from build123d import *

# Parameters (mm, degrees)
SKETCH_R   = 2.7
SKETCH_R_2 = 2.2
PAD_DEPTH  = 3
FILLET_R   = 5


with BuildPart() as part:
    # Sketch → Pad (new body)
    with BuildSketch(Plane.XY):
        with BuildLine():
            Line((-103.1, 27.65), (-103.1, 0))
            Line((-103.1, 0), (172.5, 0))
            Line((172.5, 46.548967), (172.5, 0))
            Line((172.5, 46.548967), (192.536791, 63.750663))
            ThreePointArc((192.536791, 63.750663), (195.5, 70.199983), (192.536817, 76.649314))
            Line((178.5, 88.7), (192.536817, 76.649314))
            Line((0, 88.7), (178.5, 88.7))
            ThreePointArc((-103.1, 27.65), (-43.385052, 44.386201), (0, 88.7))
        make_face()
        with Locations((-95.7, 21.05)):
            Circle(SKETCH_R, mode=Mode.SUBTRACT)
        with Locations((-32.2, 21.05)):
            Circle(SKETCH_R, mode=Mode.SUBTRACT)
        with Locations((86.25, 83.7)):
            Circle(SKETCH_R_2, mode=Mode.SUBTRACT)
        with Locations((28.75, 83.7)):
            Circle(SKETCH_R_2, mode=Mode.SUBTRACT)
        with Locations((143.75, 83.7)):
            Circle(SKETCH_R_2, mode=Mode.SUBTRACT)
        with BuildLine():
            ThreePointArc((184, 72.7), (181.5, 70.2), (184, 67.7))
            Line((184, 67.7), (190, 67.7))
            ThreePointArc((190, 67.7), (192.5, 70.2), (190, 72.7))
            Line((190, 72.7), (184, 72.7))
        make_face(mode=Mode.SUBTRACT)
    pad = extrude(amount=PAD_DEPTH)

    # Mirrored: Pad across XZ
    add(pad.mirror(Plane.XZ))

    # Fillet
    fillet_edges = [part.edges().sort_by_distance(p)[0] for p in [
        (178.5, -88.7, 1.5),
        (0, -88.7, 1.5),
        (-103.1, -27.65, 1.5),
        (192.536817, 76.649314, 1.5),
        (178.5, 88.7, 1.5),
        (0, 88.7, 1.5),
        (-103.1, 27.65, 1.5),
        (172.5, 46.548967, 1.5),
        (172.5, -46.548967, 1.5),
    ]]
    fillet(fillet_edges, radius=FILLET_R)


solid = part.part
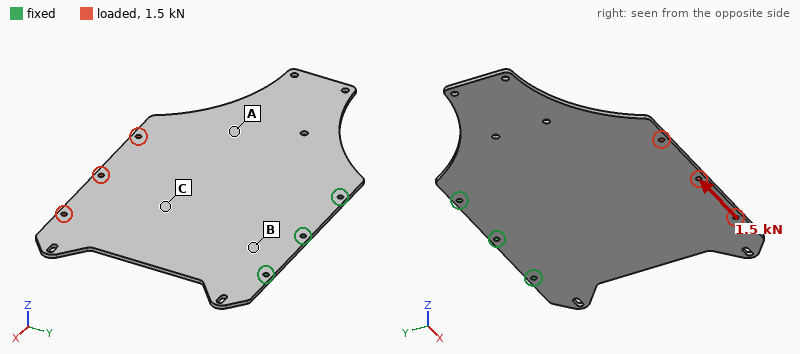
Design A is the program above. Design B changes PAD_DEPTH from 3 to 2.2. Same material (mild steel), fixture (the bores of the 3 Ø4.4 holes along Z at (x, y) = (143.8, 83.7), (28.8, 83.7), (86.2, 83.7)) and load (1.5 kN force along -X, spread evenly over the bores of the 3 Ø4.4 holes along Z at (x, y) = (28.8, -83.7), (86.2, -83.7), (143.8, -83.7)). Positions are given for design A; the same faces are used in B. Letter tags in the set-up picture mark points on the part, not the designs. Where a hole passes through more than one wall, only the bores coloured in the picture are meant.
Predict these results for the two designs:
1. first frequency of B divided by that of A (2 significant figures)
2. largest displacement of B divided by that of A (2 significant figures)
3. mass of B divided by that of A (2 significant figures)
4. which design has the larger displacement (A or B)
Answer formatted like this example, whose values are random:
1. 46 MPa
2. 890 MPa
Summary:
1. 0.74
2. 1.4
3. 0.73
4. B
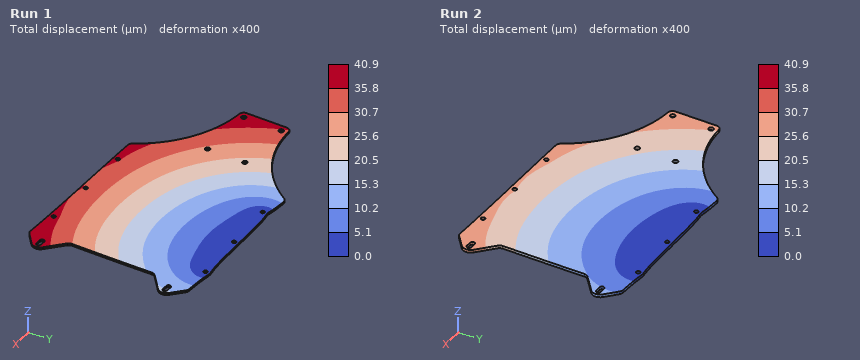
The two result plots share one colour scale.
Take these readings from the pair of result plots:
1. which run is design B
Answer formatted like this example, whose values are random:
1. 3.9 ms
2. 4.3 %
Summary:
1. Run 1
